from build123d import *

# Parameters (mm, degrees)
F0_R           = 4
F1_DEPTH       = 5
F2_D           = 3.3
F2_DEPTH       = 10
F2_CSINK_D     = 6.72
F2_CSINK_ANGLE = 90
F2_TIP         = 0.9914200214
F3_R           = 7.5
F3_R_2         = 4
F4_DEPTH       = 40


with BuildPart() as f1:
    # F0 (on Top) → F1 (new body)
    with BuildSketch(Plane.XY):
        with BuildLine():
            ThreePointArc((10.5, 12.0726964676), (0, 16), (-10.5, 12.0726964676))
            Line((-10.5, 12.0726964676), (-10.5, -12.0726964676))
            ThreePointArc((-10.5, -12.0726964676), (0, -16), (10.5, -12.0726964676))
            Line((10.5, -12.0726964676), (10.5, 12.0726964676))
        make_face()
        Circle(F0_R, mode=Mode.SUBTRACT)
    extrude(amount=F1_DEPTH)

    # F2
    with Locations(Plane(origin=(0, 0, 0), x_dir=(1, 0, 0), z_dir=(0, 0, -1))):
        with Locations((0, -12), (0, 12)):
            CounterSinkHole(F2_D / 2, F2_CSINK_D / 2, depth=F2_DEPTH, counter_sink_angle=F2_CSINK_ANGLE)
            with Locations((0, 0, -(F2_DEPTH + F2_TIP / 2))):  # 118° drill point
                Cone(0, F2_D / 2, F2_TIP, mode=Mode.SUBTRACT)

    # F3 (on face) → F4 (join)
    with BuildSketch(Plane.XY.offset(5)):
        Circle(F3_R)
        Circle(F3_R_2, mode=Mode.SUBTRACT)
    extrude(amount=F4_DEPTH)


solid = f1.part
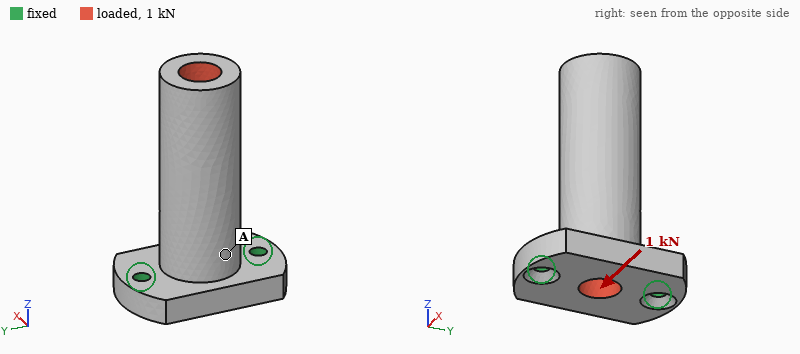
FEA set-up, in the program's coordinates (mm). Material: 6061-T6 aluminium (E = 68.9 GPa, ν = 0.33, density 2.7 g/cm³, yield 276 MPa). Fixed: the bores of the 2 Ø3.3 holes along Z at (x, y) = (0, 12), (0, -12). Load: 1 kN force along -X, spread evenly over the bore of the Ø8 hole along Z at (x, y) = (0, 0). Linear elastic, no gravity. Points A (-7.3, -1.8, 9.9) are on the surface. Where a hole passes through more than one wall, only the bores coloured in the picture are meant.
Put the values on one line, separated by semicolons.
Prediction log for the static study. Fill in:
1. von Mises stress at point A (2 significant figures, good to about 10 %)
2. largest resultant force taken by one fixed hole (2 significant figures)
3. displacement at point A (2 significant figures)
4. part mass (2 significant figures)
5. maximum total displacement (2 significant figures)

41 MPa; 500 N; 0.073 mm; 21 g; 0.34 mm
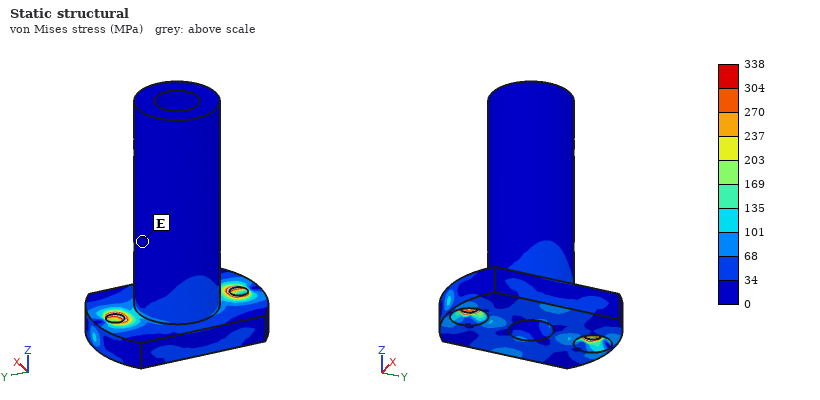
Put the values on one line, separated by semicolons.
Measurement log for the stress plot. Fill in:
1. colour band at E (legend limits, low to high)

0 to 34 MPa
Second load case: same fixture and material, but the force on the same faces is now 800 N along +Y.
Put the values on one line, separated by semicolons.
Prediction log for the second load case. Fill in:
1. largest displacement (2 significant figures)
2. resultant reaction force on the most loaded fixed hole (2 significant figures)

79 µm; 860 N
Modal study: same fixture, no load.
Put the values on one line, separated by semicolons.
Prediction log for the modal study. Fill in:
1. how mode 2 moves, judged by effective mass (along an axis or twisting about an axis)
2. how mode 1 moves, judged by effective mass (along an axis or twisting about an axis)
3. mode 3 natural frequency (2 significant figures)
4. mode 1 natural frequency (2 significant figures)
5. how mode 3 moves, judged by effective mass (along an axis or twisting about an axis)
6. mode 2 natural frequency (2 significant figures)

along Y; along X; 14 kHz; 2700 Hz; along Z; 5000 Hz
